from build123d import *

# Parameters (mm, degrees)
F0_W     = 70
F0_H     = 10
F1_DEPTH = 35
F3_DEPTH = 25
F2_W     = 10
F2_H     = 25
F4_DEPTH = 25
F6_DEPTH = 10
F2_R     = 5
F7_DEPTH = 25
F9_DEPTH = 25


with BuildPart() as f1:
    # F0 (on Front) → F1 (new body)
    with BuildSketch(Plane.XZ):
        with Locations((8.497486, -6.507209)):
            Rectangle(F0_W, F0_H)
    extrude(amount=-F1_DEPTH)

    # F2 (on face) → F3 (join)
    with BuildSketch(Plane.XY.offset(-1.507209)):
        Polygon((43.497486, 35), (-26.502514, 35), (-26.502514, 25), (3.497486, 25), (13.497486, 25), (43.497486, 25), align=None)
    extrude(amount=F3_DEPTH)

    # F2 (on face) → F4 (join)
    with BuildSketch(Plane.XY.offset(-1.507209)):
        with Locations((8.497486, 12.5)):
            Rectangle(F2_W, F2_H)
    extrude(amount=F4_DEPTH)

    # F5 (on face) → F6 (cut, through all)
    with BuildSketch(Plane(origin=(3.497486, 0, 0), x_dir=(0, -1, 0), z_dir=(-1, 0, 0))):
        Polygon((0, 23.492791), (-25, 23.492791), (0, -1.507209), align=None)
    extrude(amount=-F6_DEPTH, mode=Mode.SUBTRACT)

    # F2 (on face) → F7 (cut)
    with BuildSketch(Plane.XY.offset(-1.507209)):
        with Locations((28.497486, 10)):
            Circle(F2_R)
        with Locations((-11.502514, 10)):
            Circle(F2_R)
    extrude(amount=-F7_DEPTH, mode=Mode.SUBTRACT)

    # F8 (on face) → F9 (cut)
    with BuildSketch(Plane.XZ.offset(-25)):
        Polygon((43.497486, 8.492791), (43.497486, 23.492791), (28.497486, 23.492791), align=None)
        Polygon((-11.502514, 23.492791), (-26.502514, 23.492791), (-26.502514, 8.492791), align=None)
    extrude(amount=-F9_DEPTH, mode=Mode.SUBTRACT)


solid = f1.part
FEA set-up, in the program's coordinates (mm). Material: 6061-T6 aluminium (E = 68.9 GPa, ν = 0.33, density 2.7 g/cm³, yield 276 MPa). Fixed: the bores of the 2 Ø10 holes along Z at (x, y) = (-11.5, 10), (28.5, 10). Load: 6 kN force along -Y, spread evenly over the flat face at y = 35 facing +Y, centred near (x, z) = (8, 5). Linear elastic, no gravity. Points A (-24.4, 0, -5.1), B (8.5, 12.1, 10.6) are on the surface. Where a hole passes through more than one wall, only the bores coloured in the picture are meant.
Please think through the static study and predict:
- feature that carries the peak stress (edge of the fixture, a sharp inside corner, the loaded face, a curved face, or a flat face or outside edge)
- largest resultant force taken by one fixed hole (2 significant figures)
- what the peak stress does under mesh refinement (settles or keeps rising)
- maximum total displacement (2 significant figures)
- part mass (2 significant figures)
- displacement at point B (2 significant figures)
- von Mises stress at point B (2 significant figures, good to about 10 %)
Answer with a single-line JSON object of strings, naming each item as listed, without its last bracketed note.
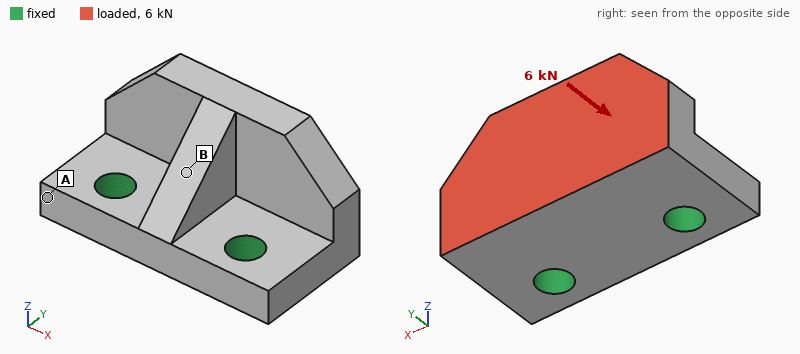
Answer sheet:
{"feature that carries the peak stress": "edge of the fixture", "largest resultant force taken by one fixed hole": "3.0 kN", "what the peak stress does under mesh refinement": "keeps rising", "maximum total displacement": "70 µm", "part mass": "110 g", "displacement at point B": "30 µm", "von Mises stress at point B": "26 MPa"}
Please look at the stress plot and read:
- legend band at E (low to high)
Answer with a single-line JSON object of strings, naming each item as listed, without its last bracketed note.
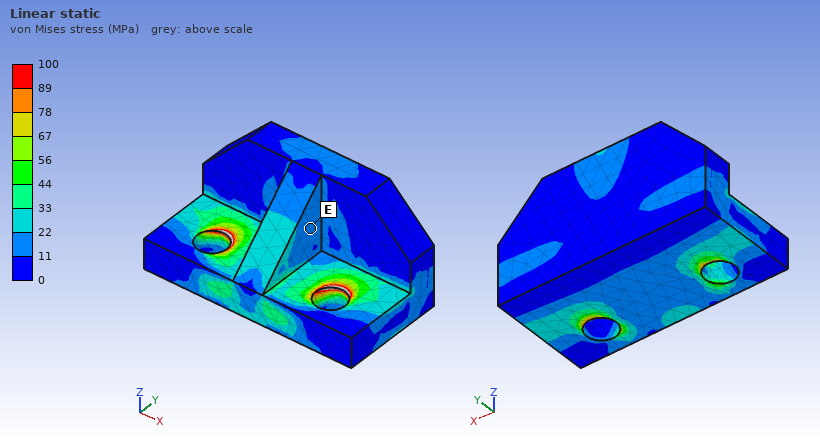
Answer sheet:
{"legend band at E": "11 to 22 MPa"}
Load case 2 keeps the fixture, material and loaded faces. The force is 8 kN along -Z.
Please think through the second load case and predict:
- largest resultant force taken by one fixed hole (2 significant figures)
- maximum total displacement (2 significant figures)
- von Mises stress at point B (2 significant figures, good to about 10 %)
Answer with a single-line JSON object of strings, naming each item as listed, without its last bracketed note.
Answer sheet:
{"largest resultant force taken by one fixed hole": "4.0 kN", "maximum total displacement": "0.14 mm", "von Mises stress at point B": "36 MPa"}
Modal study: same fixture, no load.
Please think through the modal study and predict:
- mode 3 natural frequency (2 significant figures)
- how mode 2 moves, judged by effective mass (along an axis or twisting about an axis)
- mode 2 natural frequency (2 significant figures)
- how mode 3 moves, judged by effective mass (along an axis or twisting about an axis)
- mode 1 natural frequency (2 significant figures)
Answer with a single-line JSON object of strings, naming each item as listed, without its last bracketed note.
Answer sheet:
{"mode 3 natural frequency": "14 kHz", "how mode 2 moves, judged by effective mass": "along X", "mode 2 natural frequency": "9200 Hz", "how mode 3 moves, judged by effective mass": "along X", "mode 1 natural frequency": "5800 Hz"}
